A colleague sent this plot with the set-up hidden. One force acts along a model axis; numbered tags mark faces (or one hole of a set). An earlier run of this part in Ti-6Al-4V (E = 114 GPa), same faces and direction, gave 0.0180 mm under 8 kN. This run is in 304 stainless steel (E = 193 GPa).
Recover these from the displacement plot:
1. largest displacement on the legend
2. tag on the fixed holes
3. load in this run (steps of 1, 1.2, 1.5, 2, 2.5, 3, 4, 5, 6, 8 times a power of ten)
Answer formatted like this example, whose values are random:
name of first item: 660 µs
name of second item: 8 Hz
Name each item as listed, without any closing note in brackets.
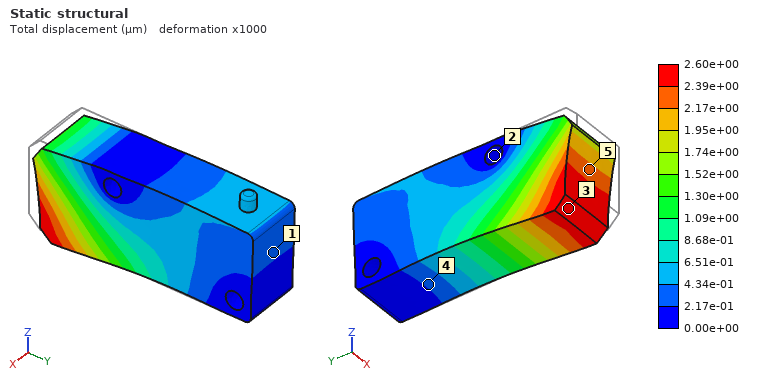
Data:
largest displacement on the legend: 2.60e+00 µm
tag on the fixed holes: 2
load in this run: 2 kN
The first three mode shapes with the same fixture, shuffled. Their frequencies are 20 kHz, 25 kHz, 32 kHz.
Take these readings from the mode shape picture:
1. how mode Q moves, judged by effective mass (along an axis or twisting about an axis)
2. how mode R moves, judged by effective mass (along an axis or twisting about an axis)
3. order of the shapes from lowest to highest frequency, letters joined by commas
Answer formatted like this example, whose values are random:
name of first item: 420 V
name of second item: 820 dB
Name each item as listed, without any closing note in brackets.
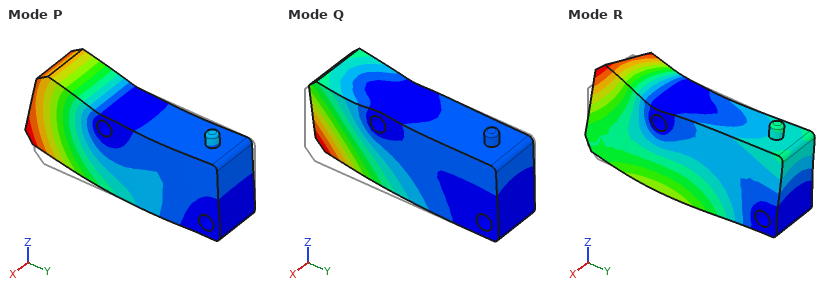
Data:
how mode Q moves, judged by effective mass: along X
how mode R moves, judged by effective mass: twisting about Y
order of the shapes from lowest to highest frequency, letters joined by commas: Q, P, R
